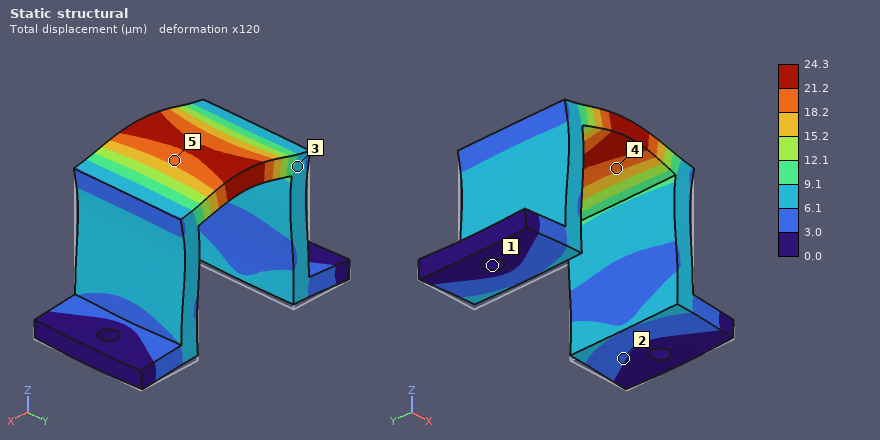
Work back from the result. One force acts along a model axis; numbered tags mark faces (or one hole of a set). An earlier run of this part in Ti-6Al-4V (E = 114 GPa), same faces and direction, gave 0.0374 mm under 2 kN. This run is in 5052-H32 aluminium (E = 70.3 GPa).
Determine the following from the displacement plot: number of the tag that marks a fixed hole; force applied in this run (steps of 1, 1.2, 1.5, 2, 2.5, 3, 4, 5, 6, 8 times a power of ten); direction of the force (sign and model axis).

1
800 N
+Z
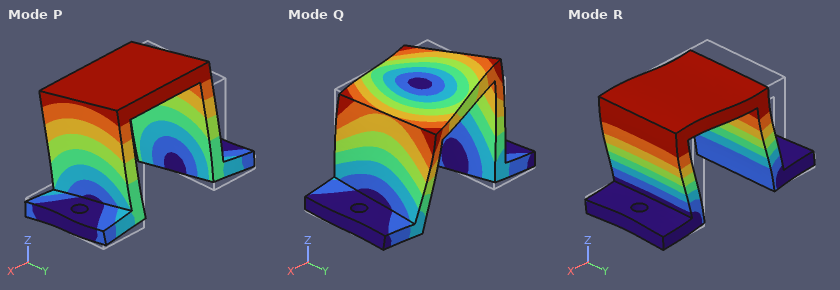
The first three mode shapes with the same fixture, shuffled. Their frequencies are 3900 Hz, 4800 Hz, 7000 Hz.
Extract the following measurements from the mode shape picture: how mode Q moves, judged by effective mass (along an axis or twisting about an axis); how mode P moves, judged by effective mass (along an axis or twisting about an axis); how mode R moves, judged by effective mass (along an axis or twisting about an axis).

twisting about Z
along Y
along X
